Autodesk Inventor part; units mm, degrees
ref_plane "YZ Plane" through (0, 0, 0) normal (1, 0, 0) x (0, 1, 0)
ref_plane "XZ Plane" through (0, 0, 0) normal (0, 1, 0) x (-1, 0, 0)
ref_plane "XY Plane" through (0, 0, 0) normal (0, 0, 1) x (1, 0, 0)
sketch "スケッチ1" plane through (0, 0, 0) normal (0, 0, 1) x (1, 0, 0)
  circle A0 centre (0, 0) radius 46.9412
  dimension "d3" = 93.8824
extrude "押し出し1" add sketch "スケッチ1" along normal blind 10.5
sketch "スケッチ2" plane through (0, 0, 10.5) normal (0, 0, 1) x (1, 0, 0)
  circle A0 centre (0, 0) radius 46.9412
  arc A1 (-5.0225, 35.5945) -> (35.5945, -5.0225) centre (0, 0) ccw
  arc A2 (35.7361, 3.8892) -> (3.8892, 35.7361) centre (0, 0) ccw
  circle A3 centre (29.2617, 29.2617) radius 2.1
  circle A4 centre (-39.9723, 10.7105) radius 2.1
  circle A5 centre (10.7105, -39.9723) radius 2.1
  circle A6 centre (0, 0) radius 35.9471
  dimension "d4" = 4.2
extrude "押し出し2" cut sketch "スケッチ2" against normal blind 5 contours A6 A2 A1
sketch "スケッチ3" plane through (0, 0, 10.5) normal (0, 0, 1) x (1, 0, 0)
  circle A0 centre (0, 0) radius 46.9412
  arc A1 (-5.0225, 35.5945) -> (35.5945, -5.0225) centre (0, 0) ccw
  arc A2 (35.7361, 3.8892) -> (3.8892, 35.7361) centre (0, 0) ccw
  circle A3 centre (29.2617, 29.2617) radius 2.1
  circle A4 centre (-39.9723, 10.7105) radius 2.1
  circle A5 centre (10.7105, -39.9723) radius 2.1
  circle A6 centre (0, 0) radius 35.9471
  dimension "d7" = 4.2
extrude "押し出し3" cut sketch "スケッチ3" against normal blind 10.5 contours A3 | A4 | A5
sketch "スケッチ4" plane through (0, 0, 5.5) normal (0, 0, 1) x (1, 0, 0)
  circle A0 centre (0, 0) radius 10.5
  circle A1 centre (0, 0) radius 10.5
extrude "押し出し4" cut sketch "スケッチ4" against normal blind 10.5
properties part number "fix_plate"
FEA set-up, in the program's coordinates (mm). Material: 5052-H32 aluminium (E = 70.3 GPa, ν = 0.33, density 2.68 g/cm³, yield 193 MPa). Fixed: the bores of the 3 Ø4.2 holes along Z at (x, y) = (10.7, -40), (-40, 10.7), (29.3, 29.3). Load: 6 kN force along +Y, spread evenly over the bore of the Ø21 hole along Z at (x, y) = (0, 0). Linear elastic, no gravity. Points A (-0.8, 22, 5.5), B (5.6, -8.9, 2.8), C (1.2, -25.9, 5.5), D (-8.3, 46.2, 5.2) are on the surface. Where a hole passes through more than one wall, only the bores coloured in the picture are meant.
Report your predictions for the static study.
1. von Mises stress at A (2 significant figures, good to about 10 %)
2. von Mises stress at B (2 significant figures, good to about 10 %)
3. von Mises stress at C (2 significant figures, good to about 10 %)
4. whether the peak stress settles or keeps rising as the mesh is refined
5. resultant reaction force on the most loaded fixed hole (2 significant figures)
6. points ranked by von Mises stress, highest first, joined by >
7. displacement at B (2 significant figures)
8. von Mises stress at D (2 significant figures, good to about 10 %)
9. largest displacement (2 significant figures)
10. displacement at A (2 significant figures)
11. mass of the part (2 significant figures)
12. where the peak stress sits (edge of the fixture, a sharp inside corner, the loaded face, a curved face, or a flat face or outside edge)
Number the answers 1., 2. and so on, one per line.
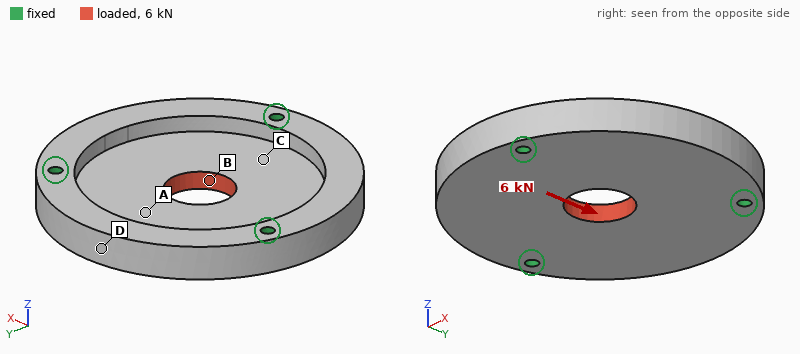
1. 13 MPa
2. 24 MPa
3. 17 MPa
4. keeps rising
5. 2.0 kN
6. B > C > A > D
7. 8.3 µm
8. 7.7 MPa
9. 12 µm
10. 8.9 µm
11. 130 g
12. edge of the fixture
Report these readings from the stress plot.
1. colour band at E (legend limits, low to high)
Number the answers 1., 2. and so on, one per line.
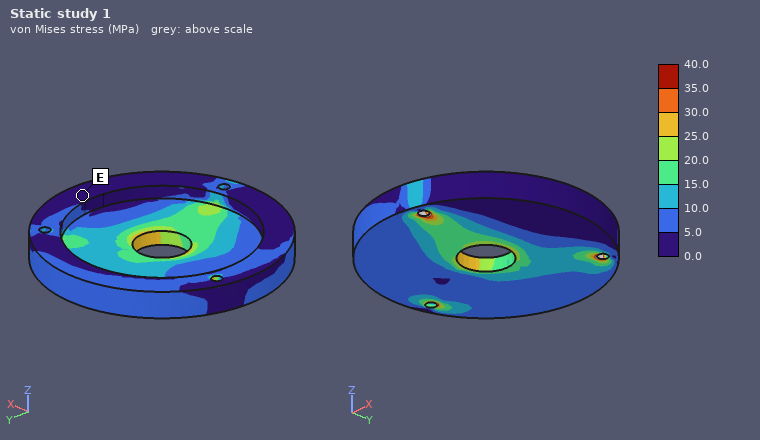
1. 0.0 to 5.0 MPa
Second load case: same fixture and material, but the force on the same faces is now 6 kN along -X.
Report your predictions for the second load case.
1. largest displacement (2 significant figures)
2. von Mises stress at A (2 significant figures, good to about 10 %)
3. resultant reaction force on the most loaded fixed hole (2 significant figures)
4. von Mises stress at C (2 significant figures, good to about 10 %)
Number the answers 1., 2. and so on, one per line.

1. 12 µm
2. 9.8 MPa
3. 2.0 kN
4. 8.1 MPa
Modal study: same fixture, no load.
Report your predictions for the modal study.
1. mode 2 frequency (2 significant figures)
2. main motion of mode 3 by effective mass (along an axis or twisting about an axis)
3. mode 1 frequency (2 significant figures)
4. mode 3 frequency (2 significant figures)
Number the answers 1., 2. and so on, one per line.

1. 5900 Hz
2. along Z
3. 5900 Hz
4. 6200 Hz
